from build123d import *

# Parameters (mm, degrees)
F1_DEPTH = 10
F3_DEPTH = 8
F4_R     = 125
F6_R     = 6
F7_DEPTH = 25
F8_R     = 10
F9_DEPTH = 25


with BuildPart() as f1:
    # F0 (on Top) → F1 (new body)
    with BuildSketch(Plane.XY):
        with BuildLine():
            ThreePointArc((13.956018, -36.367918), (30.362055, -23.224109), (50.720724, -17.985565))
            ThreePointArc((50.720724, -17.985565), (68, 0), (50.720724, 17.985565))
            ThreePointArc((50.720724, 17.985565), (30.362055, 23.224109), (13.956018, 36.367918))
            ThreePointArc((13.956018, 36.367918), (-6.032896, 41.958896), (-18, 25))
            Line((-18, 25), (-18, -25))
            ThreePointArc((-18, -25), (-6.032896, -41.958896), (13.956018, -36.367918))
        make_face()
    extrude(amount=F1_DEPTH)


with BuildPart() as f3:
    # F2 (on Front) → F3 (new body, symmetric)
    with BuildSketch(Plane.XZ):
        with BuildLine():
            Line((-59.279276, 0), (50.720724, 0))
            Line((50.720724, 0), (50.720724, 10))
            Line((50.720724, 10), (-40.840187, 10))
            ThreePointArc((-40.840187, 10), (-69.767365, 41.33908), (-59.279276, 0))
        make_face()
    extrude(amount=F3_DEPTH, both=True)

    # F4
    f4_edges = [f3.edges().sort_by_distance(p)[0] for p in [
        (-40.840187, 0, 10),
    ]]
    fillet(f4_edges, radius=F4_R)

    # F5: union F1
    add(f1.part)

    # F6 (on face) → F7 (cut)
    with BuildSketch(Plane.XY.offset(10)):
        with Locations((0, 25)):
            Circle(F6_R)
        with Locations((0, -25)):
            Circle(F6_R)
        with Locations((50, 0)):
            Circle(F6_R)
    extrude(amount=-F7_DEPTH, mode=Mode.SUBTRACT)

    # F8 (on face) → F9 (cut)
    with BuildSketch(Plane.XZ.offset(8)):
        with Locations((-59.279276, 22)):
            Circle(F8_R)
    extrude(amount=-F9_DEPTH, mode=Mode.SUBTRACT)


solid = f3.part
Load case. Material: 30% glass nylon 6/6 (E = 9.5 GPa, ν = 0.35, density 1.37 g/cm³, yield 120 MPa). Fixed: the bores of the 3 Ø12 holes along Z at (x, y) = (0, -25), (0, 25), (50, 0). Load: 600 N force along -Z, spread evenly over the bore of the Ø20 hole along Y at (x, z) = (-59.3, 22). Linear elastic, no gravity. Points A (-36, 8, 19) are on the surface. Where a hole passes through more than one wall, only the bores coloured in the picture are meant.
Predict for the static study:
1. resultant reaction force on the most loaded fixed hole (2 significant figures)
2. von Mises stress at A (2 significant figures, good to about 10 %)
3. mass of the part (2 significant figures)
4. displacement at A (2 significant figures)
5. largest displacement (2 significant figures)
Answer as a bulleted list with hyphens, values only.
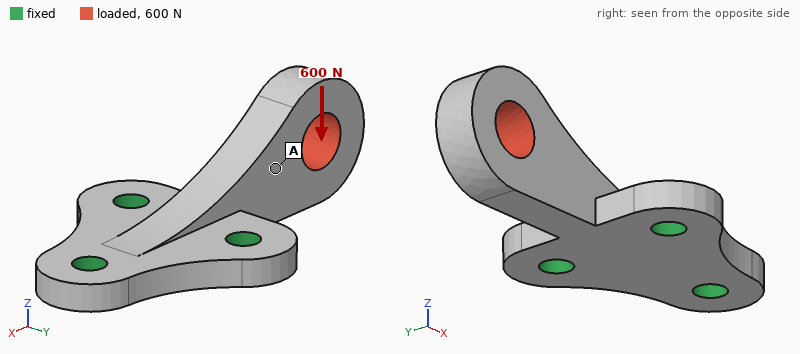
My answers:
- 590 N
- 4.9 MPa
- 110 g
- 0.36 mm
- 0.92 mm
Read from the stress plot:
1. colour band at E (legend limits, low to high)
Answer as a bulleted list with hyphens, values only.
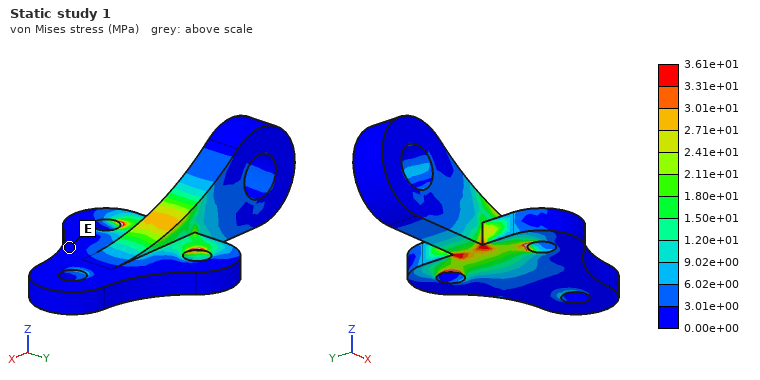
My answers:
- 0.00e+00 to 3.01e+00 MPa
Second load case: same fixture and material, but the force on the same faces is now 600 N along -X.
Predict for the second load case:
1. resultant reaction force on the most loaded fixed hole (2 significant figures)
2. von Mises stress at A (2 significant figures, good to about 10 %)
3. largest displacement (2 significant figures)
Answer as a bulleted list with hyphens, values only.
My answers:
- 220 N
- 1.8 MPa
- 0.26 mm
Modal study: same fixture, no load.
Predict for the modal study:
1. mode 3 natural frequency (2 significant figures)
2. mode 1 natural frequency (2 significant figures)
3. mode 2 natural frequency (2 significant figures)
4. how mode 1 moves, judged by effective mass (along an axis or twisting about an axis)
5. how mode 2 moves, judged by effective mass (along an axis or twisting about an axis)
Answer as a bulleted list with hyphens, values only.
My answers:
- 2800 Hz
- 830 Hz
- 1100 Hz
- along Z
- along Y
